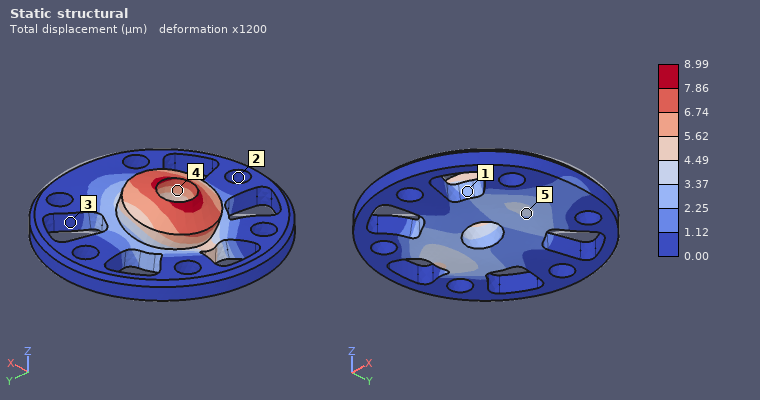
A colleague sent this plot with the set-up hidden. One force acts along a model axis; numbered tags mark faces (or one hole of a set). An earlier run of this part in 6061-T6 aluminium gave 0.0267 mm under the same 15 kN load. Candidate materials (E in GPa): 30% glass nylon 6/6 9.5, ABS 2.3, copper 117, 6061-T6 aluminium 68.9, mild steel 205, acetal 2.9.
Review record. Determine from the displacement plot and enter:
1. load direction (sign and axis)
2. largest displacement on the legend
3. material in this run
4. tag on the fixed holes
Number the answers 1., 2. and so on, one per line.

1. -X
2. 8.99 µm
3. mild steel
4. 2
